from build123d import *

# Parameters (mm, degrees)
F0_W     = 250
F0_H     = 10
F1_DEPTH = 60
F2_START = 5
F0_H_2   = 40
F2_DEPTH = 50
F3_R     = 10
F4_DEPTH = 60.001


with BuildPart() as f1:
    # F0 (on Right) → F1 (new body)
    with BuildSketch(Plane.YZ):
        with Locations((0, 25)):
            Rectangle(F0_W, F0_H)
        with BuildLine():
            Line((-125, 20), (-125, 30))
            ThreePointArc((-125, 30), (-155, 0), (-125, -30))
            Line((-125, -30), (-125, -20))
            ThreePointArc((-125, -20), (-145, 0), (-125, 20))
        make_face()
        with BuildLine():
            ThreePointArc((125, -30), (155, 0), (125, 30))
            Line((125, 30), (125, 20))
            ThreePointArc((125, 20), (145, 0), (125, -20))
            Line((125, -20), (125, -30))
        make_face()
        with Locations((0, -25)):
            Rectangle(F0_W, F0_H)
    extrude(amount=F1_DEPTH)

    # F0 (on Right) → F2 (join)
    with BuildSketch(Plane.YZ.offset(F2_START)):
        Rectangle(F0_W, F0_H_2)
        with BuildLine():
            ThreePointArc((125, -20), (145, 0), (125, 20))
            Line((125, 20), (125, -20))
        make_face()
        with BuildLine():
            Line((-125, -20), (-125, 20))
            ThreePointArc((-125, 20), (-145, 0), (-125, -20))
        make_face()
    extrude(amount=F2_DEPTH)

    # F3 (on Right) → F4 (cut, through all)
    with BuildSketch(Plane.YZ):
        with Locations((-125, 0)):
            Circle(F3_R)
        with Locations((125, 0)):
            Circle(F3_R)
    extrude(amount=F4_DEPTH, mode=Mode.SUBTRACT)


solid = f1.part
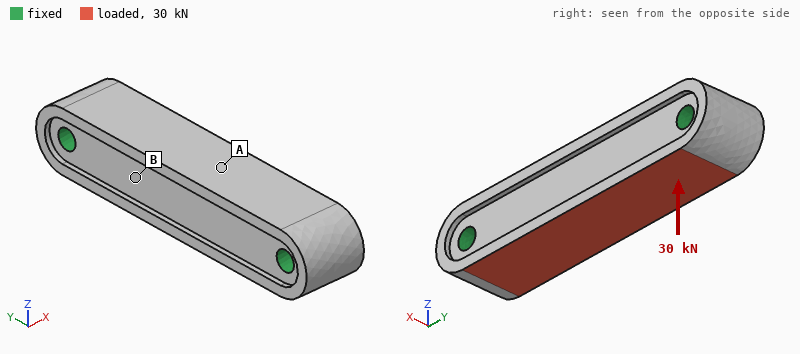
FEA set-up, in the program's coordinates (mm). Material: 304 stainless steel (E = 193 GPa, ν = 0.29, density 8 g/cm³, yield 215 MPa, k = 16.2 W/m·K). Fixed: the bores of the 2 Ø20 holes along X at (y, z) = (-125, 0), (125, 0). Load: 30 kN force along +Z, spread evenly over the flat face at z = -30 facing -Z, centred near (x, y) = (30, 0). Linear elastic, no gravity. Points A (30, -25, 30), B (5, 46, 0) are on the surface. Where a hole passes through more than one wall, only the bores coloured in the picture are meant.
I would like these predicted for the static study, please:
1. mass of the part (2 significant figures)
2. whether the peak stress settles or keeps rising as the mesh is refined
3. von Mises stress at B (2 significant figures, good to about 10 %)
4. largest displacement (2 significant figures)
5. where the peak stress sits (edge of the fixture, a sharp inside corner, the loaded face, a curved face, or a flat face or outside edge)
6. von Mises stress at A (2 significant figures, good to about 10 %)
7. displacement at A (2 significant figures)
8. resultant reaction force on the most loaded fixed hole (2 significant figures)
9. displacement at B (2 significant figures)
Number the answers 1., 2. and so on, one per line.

1. 7.4 kg
2. keeps rising
3. 5.4 MPa
4. 15 µm
5. edge of the fixture
6. 12 MPa
7. 14 µm
8. 15 kN
9. 12 µm
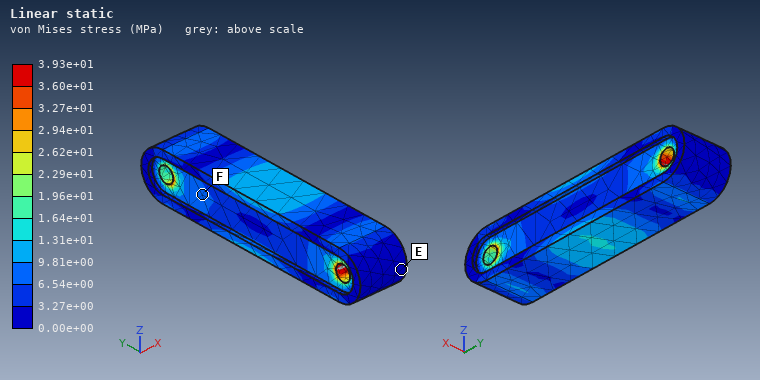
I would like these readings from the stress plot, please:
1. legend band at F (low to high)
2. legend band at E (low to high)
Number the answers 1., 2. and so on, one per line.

1. 6.54e+00 to 9.81e+00 MPa
2. 0.00e+00 to 3.27e+00 MPa
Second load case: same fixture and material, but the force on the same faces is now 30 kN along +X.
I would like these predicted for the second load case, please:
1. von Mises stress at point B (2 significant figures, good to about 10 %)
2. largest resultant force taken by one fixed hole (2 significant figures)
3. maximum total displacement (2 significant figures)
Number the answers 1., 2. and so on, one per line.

1. 11 MPa
2. 15 kN
3. 24 µm
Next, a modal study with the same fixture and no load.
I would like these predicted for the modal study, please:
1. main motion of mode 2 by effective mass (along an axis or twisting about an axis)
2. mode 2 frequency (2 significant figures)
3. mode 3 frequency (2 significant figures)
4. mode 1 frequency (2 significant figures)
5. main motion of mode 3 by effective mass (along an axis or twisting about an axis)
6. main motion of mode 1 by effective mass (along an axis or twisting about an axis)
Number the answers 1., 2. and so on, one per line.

1. along X
2. 3400 Hz
3. 5200 Hz
4. 3100 Hz
5. twisting about Y
6. along Z
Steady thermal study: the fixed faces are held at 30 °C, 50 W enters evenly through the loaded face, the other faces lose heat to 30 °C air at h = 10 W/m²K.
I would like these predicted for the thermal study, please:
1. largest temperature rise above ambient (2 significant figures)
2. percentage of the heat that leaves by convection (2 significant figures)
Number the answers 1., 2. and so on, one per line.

1. 29 K
2. 16 %
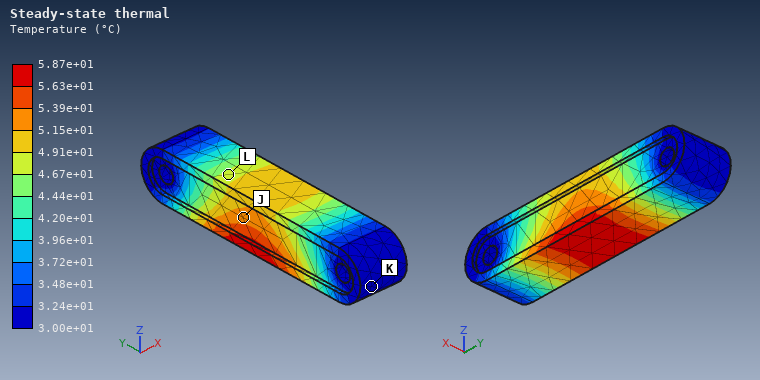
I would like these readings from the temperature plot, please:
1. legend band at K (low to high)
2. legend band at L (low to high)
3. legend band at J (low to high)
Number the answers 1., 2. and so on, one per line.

1. 3.00e+01 to 3.24e+01 °C
2. 4.67e+01 to 4.91e+01 °C
3. 5.15e+01 to 5.39e+01 °C
